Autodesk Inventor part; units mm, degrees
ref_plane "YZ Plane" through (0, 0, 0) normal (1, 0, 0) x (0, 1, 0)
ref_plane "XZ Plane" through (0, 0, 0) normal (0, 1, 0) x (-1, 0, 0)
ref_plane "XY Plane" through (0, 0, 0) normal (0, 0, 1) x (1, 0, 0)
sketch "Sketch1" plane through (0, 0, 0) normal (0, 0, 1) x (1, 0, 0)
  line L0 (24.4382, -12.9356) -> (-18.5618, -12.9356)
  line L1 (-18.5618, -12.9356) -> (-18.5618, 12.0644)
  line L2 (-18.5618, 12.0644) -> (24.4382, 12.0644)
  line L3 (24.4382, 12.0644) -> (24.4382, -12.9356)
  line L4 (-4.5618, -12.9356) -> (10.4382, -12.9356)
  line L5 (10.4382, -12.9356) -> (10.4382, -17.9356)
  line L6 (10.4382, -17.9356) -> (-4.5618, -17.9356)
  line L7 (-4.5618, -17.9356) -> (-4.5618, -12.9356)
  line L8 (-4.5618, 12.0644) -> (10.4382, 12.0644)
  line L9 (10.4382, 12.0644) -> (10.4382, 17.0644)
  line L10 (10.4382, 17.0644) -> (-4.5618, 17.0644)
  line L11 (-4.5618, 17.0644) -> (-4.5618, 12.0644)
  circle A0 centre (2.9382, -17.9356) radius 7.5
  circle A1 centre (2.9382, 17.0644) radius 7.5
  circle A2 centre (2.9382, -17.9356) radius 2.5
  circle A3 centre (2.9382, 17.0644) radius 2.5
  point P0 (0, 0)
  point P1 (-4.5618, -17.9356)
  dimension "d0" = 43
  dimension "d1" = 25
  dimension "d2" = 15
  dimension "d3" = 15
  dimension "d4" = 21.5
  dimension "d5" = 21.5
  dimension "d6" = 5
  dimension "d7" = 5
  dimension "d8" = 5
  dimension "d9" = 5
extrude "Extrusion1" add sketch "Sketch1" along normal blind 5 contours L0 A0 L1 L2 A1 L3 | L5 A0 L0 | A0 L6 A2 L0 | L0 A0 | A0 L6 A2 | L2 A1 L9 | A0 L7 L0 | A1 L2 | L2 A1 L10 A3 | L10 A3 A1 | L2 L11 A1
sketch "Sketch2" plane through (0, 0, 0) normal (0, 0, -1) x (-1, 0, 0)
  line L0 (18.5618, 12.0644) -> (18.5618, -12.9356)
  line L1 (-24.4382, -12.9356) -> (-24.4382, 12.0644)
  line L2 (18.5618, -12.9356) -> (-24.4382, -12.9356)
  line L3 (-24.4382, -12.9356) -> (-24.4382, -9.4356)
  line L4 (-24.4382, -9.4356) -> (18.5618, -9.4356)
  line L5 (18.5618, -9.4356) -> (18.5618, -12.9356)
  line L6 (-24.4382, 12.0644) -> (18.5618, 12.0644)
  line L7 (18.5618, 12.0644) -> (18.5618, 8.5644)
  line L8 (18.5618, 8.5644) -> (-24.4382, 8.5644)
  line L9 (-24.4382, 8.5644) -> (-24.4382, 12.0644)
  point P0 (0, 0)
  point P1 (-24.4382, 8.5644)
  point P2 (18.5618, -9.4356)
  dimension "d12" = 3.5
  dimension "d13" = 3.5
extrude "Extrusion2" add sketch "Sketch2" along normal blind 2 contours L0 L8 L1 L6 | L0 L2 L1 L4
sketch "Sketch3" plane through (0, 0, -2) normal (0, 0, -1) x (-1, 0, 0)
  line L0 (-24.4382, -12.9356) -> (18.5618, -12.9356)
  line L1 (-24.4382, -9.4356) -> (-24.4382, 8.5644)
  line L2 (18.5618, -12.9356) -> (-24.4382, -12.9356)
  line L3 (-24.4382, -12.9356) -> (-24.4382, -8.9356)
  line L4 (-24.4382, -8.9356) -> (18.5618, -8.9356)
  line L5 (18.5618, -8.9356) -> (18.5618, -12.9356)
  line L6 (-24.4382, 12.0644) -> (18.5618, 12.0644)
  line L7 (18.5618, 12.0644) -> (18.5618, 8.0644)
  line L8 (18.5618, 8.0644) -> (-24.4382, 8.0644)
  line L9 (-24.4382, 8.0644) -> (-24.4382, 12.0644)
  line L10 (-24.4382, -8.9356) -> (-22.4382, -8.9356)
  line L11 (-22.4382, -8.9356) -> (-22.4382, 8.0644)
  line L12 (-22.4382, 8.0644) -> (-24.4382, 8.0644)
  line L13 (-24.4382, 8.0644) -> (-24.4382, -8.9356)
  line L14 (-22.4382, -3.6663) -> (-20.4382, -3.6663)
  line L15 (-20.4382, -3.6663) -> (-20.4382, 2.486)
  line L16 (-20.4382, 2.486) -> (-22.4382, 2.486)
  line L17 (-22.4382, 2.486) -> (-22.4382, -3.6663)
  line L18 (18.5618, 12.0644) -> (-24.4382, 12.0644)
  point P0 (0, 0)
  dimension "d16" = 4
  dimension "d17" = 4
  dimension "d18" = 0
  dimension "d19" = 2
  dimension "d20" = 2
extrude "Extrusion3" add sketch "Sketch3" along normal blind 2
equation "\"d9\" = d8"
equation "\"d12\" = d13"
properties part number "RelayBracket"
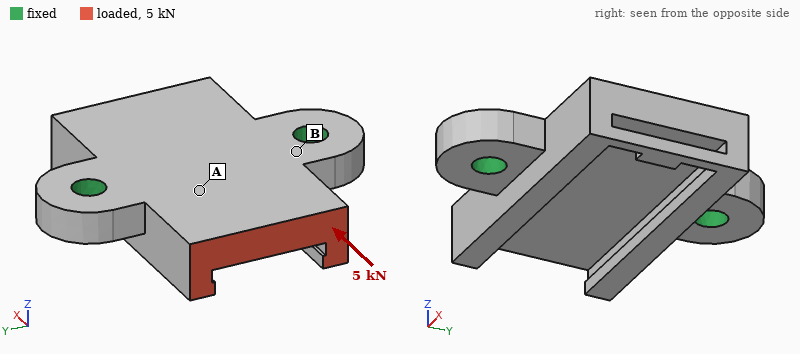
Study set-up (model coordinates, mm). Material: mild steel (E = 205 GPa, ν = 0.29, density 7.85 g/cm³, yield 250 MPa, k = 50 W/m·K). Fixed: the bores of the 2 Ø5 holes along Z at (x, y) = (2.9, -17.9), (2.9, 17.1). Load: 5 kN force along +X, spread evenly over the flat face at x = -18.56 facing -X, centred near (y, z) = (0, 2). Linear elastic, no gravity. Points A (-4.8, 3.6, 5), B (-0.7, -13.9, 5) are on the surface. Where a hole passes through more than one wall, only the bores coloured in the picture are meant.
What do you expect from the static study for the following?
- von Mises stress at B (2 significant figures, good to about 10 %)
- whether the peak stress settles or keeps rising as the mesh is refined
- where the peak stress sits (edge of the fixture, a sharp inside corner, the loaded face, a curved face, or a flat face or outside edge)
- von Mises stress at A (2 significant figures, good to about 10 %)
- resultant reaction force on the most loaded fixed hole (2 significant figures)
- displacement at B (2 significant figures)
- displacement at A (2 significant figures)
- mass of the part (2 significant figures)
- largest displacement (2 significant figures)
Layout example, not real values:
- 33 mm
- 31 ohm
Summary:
- 54 MPa
- keeps rising
- edge of the fixture
- 21 MPa
- 2.5 kN
- 1.4 µm
- 4.1 µm
- 64 g
- 9.3 µm
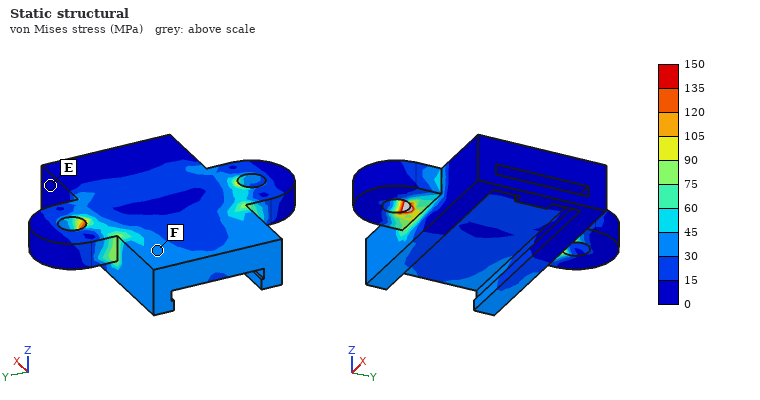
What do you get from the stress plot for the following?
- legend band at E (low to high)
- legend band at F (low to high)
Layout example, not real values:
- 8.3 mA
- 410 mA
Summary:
- 0 to 15 MPa
- 30 to 45 MPa
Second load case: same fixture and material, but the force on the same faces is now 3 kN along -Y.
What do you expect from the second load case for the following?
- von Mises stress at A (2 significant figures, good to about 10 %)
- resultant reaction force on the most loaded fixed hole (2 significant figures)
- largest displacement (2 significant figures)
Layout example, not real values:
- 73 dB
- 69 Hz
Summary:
- 25 MPa
- 2.4 kN
- 20 µm
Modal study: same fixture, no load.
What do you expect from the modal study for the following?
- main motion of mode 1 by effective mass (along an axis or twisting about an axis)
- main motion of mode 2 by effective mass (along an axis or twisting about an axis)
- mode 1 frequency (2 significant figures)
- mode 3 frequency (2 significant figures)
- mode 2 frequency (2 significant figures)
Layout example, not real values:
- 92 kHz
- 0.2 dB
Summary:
- twisting about Y
- along Z
- 6600 Hz
- 16 kHz
- 11 kHz
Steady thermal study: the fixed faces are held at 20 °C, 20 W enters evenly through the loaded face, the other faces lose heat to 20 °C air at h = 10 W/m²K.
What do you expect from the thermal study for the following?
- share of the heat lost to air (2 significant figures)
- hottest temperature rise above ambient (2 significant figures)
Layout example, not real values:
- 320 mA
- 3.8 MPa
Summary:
- 4.5 %
- 64 K
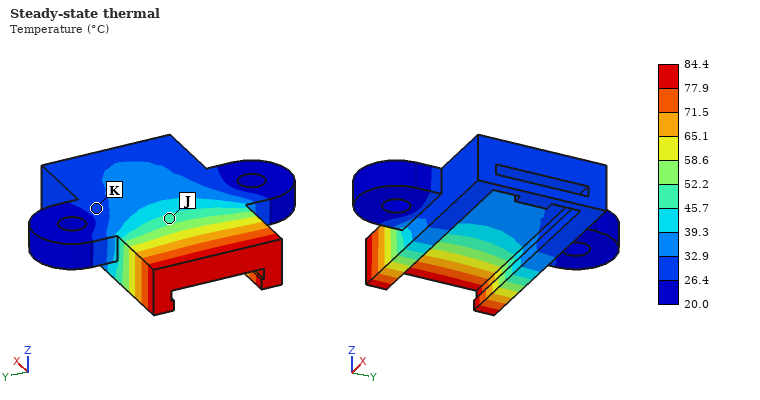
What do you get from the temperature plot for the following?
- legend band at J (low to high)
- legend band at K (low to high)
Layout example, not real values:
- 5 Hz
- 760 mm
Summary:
- 45.7 to 52.2 °C
- 26.4 to 32.9 °C
